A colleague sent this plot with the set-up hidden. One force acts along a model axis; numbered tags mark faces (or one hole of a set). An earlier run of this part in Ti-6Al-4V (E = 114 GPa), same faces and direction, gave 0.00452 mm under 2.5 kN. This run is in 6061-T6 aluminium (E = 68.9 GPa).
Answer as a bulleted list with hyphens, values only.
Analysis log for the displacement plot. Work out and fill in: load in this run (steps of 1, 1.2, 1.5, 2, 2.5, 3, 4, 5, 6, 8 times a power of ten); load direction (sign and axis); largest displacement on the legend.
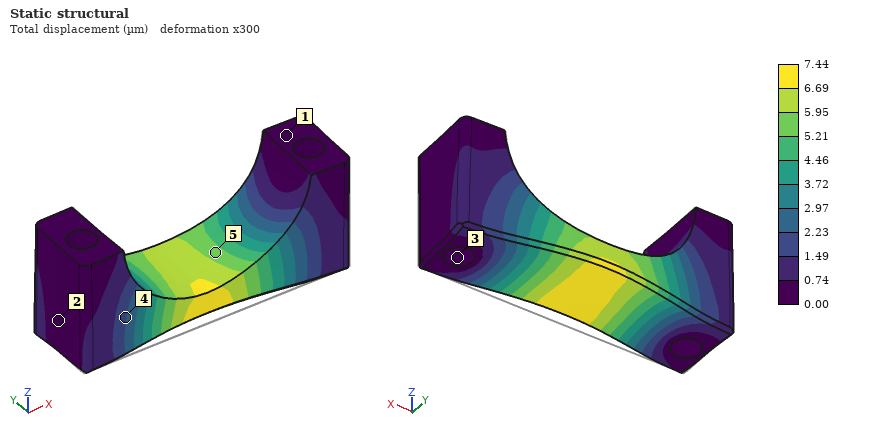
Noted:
- 2.5 kN
- +Y
- 7.44 µm
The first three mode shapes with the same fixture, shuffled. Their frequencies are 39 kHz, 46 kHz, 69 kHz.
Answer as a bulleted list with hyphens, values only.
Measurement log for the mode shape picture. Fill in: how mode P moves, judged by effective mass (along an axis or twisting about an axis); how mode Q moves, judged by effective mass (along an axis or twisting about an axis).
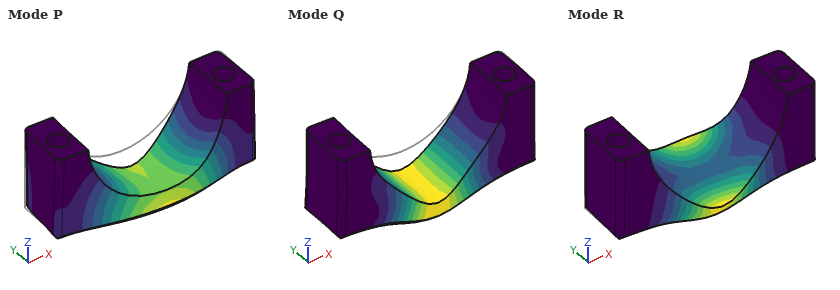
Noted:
- along Y
- along Z
